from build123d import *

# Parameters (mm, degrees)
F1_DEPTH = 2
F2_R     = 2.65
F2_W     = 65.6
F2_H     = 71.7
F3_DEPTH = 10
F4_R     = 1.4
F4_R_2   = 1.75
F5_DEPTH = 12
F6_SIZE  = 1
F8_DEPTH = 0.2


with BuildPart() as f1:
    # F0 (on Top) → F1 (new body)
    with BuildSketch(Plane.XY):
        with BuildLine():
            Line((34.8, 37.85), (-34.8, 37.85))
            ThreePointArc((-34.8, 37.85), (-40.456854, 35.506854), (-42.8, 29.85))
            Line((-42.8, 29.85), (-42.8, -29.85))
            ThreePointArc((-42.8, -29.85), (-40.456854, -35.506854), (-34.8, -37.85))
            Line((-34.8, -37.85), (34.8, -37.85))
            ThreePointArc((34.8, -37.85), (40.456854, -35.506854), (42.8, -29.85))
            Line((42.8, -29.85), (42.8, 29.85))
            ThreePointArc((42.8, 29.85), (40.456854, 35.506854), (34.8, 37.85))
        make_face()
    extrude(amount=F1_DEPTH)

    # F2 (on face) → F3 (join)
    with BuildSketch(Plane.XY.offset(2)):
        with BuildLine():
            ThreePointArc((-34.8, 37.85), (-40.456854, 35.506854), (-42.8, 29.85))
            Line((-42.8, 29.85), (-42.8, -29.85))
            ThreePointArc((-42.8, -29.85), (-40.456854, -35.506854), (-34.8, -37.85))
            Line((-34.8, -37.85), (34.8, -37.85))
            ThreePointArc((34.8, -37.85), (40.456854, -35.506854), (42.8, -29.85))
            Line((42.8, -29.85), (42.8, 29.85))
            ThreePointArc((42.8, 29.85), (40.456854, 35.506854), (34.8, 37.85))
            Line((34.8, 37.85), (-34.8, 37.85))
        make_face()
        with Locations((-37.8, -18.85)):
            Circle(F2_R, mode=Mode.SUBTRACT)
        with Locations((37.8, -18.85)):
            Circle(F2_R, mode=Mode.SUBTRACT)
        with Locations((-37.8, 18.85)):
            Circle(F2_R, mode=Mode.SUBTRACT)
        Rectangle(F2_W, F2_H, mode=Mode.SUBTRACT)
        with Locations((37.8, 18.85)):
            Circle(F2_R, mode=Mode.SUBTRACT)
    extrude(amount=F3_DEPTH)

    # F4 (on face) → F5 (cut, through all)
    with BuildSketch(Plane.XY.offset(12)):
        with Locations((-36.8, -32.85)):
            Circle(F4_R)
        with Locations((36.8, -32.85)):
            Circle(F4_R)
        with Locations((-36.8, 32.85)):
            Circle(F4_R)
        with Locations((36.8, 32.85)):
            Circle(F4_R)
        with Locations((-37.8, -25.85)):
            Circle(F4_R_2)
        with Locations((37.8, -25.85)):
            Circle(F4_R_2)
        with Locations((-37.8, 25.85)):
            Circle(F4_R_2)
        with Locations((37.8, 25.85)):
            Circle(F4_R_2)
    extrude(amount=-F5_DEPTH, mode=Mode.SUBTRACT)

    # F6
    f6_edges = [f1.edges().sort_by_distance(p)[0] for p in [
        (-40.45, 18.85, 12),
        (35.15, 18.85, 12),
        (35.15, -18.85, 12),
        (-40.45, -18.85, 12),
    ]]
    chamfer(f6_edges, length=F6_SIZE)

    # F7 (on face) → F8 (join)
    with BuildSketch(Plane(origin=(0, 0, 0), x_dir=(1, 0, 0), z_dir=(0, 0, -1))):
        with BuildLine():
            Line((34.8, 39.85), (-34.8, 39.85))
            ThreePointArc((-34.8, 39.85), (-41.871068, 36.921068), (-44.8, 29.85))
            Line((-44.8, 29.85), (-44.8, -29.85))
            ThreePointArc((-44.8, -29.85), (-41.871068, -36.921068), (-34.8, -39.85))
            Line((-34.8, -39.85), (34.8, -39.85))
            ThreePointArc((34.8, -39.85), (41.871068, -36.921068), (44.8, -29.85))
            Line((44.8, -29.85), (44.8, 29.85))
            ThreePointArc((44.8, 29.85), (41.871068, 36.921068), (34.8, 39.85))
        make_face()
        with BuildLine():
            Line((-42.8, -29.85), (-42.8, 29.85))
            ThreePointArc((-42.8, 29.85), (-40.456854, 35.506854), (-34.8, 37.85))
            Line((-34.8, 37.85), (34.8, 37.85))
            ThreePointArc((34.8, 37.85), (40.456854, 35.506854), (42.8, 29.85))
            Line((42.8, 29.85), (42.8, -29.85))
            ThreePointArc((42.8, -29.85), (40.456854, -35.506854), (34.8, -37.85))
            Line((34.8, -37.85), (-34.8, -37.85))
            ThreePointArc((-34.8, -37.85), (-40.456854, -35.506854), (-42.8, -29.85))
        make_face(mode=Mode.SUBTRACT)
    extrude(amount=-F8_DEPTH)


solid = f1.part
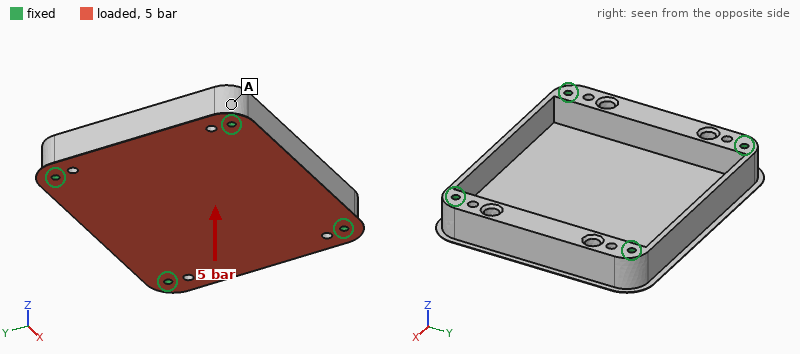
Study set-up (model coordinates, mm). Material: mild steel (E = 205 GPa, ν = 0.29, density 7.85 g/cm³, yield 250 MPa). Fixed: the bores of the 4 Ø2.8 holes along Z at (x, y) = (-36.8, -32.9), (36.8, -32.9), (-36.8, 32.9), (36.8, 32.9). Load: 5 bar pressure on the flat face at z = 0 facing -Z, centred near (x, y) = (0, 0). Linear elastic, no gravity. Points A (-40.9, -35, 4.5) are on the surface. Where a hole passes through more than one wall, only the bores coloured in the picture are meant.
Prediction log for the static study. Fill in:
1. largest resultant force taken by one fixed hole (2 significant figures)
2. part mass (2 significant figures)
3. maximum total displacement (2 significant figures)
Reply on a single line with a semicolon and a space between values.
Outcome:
960 N; 220 g; 0.14 mm
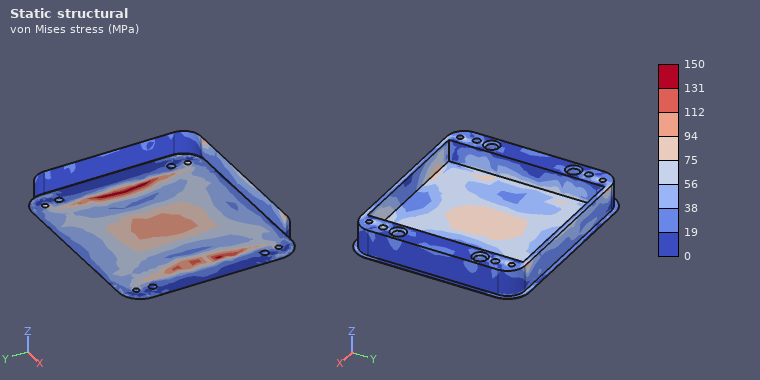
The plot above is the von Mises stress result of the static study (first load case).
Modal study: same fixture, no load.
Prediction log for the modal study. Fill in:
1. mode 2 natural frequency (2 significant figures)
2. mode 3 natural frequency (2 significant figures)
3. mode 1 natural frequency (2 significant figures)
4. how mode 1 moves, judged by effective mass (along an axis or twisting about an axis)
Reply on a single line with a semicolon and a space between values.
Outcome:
5000 Hz; 6700 Hz; 2900 Hz; along Z
